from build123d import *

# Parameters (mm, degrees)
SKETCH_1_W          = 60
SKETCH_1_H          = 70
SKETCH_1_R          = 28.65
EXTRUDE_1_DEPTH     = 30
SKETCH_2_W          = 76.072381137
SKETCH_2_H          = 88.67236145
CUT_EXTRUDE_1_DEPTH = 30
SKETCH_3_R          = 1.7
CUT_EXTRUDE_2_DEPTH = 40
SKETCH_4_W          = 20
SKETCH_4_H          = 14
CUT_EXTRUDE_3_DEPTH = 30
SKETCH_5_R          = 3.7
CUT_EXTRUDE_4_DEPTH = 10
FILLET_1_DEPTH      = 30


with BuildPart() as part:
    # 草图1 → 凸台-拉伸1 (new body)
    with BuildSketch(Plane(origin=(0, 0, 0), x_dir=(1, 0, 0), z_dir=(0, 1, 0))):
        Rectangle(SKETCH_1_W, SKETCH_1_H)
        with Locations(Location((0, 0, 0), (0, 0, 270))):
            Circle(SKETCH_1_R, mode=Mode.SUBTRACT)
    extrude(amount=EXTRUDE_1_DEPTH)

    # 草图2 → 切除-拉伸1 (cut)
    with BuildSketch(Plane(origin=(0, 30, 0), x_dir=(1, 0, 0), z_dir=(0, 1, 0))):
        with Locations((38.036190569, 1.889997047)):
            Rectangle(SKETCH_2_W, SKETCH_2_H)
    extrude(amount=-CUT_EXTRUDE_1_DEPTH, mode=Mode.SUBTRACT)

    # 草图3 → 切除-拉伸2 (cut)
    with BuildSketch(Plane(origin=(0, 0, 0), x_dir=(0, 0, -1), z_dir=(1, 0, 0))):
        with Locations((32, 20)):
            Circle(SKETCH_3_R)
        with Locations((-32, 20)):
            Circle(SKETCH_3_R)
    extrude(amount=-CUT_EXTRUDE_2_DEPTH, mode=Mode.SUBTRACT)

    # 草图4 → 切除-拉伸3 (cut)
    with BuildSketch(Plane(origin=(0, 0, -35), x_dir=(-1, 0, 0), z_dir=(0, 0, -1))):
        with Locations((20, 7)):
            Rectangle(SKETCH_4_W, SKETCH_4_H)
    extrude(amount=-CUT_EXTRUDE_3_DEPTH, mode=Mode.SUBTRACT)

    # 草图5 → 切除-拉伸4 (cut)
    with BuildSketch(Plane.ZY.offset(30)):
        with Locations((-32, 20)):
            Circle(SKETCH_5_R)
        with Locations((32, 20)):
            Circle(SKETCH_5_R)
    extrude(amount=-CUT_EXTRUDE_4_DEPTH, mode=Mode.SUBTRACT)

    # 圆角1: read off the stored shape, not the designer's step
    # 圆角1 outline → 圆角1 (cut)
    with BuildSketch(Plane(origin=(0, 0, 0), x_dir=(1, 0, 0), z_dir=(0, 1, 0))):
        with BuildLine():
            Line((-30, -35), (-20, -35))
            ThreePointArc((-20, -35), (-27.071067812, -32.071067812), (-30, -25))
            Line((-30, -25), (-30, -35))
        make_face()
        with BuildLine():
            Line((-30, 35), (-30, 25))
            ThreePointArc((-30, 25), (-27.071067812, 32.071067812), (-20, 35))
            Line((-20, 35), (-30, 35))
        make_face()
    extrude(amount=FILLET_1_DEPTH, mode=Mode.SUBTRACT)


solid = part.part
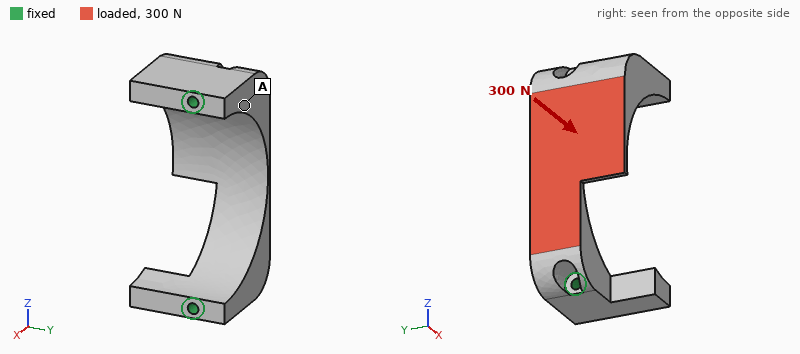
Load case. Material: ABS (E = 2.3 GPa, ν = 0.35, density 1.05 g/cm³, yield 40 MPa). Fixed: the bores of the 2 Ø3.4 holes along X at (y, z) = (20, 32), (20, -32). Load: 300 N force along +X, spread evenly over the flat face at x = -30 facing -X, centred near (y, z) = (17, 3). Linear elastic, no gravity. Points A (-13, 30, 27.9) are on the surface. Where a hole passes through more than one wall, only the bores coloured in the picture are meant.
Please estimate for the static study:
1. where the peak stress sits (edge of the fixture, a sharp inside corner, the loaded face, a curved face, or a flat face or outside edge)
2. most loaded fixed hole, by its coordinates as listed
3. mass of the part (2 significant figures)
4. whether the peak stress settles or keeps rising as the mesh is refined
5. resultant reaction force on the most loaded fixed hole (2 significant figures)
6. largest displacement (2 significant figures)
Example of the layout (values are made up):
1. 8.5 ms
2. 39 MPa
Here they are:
1. a sharp inside corner
2. (20, 32)
3. 19 g
4. keeps rising
5. 240 N
6. 0.90 mm
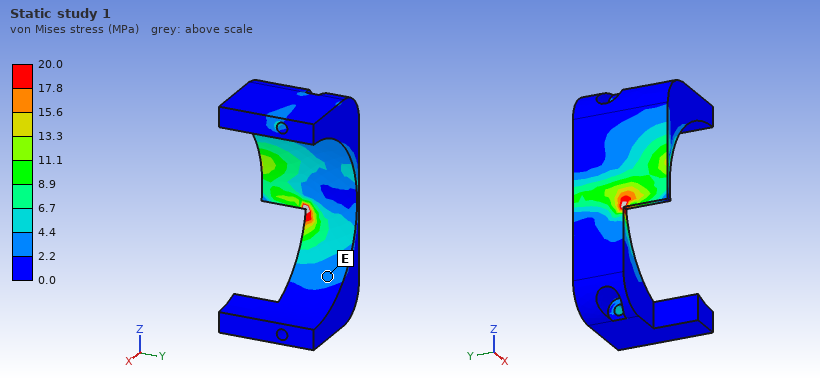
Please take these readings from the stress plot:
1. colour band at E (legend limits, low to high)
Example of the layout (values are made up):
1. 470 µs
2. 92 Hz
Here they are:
1. 2.2 to 4.4 MPa
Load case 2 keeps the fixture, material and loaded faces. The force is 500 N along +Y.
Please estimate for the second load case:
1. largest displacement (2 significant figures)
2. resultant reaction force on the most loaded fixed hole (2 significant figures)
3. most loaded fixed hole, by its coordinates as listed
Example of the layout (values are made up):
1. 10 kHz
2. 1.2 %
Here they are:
1. 0.61 mm
2. 290 N
3. (20, 32)
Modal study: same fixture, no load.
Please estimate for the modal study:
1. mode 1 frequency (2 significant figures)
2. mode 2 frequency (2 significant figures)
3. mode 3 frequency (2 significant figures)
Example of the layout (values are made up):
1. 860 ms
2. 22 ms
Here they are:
1. 2600 Hz
2. 2900 Hz
3. 3600 Hz
